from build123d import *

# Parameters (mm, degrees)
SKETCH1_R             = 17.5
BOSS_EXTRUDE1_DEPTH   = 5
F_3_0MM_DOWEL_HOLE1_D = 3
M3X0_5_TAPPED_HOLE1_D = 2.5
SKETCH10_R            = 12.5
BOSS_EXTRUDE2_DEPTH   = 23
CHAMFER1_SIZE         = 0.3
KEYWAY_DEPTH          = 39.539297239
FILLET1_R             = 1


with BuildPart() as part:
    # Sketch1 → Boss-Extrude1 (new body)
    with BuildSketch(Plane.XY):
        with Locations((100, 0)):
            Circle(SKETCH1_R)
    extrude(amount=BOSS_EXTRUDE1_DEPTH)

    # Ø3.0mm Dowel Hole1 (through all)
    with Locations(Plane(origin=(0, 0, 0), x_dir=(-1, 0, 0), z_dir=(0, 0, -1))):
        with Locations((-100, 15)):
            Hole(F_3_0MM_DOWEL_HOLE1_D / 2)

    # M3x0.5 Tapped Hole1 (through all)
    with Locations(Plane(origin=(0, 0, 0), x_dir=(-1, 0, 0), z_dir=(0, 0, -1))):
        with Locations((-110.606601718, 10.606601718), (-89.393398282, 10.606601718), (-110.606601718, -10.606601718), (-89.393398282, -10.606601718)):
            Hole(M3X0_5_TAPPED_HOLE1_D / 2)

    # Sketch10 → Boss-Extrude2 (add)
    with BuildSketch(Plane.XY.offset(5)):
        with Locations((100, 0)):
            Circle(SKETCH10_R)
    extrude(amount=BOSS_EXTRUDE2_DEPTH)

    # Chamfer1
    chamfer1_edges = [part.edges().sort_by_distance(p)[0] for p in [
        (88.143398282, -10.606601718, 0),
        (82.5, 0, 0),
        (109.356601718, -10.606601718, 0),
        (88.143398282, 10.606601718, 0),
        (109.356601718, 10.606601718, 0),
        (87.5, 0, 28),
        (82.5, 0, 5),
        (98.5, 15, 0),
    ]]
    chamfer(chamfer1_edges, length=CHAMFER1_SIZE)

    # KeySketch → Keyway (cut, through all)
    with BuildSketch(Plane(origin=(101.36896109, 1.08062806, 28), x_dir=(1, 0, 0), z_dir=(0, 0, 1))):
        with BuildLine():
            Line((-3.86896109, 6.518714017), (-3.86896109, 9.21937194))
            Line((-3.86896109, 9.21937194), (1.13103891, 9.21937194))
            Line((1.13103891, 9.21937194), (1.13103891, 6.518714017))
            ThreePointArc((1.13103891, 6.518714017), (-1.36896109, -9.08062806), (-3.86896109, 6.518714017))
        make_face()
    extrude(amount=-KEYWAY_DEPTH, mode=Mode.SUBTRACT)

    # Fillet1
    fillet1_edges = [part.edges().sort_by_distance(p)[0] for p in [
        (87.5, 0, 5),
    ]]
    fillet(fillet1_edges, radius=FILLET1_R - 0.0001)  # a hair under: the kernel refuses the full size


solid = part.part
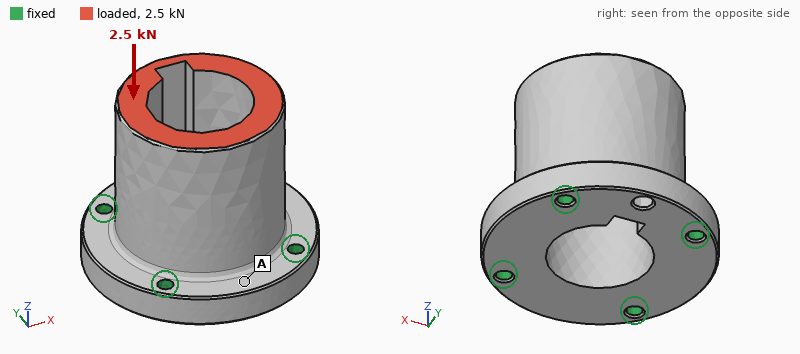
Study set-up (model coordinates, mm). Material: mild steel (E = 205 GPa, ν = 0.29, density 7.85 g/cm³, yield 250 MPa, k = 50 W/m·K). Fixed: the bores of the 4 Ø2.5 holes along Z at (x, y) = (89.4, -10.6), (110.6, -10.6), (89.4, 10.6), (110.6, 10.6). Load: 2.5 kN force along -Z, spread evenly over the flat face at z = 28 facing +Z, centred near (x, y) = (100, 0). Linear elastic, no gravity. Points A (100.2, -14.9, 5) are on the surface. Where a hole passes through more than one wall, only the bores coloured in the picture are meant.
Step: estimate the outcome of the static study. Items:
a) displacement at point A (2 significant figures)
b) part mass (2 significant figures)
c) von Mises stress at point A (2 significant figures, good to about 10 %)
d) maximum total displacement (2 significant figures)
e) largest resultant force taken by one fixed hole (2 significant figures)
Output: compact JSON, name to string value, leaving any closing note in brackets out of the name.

{"displacement at point A": "1.0 µm", "part mass": "78 g", "von Mises stress at point A": "8.3 MPa", "maximum total displacement": "2.1 µm", "largest resultant force taken by one fixed hole": "680 N"}
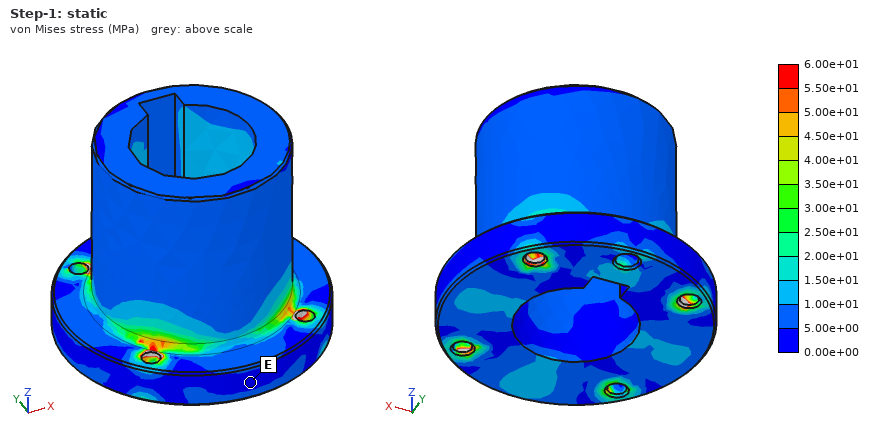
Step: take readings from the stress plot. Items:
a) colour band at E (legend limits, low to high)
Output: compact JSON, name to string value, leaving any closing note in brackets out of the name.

{"colour band at E": "0.00e+00 to 5.00e+00 MPa"}
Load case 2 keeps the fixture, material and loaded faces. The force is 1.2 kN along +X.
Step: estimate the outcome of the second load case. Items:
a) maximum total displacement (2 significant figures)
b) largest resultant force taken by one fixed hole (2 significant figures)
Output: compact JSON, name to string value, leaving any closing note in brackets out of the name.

{"maximum total displacement": "8.9 µm", "largest resultant force taken by one fixed hole": "840 N"}
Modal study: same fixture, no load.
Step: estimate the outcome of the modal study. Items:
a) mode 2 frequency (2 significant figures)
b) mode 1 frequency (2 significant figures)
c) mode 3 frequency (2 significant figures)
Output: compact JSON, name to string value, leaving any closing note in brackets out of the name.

{"mode 2 frequency": "15 kHz", "mode 1 frequency": "14 kHz", "mode 3 frequency": "24 kHz"}
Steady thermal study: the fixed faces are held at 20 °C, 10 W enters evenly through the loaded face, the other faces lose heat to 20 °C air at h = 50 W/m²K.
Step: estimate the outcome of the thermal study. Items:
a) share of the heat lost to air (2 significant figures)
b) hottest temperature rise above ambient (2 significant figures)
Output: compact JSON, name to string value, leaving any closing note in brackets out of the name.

{"share of the heat lost to air": "19 %", "hottest temperature rise above ambient": "19 K"}
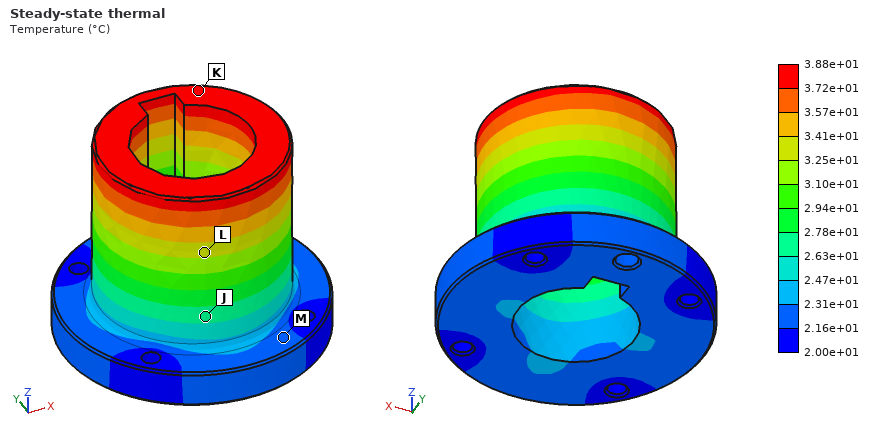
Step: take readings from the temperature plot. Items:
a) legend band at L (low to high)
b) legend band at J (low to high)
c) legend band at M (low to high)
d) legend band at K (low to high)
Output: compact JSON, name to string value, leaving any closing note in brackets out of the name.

{"legend band at L": "3.25e+01 to 3.41e+01 °C", "legend band at J": "2.63e+01 to 2.78e+01 °C", "legend band at M": "2.16e+01 to 2.31e+01 °C", "legend band at K": "3.72e+01 to 3.88e+01 °C"}
